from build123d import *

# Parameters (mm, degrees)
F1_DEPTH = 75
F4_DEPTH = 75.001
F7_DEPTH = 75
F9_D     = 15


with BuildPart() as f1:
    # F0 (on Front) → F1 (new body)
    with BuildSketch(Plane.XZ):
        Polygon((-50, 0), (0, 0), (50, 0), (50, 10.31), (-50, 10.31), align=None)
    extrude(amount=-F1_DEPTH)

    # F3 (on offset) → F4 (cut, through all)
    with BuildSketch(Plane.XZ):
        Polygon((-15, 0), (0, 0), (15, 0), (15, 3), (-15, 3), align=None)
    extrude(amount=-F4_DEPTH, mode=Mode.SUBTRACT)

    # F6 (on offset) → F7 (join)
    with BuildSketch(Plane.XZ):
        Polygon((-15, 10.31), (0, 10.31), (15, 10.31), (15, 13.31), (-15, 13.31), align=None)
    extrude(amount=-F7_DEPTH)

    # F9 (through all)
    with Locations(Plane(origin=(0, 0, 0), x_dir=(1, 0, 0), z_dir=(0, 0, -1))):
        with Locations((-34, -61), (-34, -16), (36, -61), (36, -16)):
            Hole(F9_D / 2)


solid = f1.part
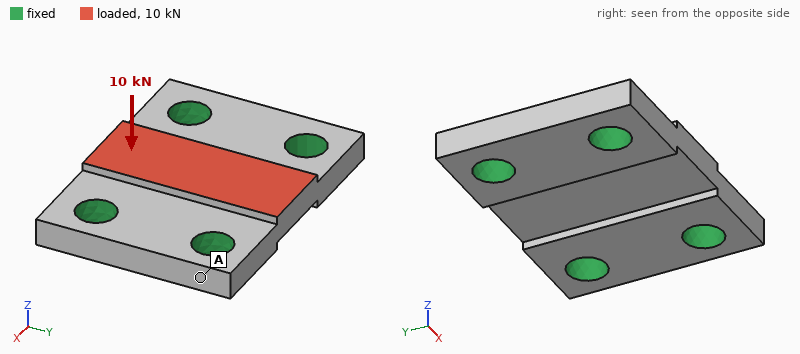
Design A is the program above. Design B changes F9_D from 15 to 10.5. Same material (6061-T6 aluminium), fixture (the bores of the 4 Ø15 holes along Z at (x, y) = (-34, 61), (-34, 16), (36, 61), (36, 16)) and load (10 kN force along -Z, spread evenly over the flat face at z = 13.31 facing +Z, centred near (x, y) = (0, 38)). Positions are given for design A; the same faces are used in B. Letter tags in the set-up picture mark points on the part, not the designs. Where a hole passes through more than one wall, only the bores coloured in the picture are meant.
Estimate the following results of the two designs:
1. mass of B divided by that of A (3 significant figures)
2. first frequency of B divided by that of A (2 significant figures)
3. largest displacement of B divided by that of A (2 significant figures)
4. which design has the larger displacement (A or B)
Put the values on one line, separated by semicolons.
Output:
1.05; 0.85; 1.3; B
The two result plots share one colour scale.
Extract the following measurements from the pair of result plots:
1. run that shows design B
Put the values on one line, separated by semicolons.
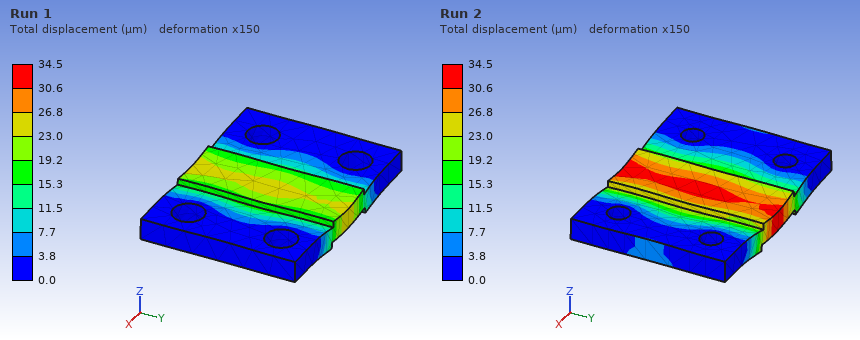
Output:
Run 2
